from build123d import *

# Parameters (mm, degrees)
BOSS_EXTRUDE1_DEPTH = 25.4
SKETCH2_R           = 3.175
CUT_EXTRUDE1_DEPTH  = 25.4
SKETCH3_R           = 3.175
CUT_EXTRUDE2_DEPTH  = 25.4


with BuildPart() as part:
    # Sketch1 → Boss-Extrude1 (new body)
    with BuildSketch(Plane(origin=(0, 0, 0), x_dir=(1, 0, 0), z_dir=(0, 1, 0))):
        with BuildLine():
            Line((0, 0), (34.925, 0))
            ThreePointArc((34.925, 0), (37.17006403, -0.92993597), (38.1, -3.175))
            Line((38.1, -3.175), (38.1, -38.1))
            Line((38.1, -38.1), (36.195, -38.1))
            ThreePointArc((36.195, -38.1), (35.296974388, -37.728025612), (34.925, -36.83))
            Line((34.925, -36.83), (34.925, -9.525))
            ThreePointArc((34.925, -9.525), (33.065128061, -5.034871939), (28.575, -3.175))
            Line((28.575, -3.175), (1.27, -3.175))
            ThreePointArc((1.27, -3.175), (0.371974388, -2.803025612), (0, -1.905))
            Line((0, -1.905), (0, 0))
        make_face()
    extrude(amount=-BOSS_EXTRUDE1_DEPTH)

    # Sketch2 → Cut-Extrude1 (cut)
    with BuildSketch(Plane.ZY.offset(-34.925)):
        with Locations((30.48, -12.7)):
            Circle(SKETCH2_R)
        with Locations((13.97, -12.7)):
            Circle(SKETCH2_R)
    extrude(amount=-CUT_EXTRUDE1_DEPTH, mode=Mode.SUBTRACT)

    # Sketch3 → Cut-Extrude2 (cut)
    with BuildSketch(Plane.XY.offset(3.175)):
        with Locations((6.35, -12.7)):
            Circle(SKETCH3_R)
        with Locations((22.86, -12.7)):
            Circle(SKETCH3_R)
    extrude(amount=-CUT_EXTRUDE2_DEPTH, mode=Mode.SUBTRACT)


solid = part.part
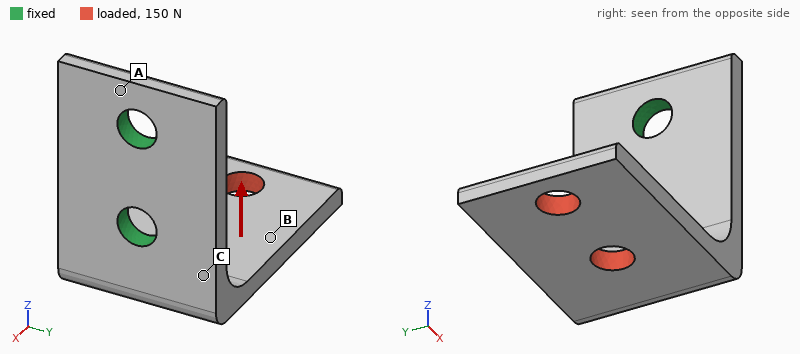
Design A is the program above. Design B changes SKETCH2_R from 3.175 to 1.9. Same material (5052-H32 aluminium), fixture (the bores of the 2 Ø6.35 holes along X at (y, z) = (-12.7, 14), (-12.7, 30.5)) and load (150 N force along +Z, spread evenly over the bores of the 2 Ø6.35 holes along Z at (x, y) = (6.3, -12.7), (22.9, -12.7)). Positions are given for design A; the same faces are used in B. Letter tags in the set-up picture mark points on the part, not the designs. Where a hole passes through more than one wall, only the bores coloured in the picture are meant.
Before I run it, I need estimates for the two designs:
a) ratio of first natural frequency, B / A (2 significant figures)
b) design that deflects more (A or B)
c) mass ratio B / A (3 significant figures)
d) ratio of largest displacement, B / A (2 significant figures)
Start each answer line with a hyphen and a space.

- 0.93
- B
- 1.02
- 1.1
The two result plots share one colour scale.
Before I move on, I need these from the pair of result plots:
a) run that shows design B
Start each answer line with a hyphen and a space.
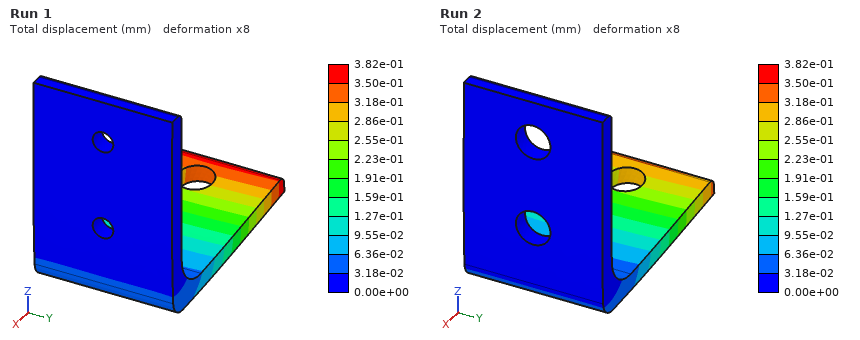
- Run 1
